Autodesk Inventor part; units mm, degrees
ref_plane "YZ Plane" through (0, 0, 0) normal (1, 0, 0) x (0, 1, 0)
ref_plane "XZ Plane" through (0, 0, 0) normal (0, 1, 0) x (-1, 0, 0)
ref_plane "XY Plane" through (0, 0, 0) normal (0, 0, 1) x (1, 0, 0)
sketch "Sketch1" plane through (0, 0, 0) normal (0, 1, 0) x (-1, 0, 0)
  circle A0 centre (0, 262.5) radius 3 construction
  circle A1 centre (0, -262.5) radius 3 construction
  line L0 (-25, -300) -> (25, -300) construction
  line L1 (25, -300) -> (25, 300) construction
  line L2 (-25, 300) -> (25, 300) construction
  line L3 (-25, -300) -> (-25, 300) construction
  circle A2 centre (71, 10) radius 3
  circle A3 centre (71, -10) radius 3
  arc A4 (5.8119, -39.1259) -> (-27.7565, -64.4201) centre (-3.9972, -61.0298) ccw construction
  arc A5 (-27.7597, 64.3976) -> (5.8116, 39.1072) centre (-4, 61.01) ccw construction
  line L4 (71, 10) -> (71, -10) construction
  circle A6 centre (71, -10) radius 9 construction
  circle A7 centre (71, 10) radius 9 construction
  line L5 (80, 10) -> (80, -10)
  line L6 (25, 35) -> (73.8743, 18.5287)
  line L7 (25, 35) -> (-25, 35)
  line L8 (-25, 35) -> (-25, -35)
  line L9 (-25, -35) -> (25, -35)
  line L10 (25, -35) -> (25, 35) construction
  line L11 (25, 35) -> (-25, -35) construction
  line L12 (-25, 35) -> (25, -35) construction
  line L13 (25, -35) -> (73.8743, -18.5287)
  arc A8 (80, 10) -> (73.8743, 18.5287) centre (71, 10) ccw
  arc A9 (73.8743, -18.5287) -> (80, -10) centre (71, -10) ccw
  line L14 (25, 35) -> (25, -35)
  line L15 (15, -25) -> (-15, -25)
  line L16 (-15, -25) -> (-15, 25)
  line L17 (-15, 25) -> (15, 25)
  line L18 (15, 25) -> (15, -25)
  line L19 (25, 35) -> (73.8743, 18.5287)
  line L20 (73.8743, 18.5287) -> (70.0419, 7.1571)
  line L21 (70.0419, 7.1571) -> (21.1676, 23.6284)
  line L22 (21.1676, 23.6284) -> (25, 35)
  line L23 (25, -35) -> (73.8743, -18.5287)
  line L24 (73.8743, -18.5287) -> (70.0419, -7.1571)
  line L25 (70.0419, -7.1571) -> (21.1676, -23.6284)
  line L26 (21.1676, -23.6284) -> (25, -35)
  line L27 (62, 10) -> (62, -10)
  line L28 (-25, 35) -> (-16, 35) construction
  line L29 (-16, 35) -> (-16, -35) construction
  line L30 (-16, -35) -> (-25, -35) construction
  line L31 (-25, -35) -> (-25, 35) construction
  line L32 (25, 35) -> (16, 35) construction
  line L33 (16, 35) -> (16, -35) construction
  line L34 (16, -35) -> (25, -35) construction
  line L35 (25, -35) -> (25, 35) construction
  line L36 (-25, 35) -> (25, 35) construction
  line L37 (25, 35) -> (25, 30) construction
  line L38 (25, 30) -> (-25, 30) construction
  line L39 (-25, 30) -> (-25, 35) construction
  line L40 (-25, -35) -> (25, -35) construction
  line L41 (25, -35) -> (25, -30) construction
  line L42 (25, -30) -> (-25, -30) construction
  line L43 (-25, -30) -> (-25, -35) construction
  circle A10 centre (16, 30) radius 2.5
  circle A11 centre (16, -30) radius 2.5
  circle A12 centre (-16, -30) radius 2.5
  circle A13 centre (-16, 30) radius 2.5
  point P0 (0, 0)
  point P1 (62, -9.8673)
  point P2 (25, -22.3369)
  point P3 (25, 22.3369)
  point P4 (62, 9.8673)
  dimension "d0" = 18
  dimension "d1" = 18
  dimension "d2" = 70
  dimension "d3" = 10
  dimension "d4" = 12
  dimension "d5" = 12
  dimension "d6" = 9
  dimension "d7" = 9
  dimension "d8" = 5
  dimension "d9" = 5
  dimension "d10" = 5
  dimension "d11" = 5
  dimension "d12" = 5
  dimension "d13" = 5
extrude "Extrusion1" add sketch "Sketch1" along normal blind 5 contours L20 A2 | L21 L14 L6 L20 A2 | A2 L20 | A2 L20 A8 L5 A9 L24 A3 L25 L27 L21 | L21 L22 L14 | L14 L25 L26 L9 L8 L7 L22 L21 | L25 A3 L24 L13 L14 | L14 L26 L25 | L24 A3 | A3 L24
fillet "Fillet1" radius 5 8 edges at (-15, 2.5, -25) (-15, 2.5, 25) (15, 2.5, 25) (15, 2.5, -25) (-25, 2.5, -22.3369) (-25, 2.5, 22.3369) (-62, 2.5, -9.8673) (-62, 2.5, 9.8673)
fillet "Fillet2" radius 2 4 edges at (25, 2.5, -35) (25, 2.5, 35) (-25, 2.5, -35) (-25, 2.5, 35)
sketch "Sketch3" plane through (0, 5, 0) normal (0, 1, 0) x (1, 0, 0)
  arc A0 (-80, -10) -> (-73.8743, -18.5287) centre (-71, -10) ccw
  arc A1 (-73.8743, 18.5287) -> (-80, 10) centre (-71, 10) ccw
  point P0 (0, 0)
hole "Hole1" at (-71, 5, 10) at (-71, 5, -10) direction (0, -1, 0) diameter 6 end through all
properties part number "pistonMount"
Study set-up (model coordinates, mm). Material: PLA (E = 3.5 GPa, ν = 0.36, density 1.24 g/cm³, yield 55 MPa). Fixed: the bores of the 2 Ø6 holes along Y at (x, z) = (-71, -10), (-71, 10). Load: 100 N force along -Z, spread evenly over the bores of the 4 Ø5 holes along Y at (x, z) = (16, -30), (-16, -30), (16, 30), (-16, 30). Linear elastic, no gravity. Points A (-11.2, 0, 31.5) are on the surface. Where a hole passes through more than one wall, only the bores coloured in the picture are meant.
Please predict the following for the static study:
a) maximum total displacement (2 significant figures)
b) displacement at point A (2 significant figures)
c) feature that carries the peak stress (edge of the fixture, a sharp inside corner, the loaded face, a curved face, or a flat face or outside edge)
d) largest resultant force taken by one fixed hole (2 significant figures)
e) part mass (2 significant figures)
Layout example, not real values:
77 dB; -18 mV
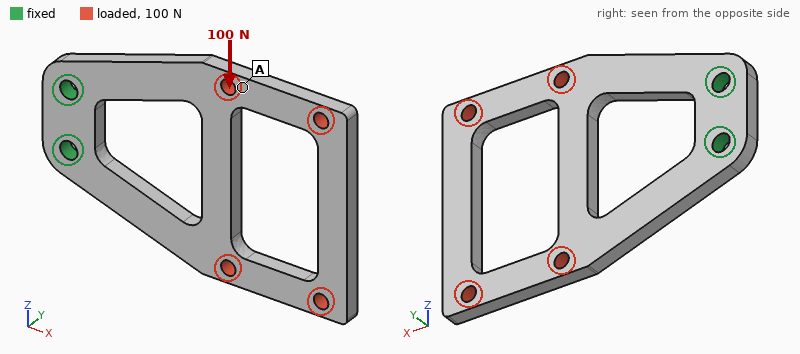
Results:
1.3 mm; 0.79 mm; a curved face; 220 N; 22 g
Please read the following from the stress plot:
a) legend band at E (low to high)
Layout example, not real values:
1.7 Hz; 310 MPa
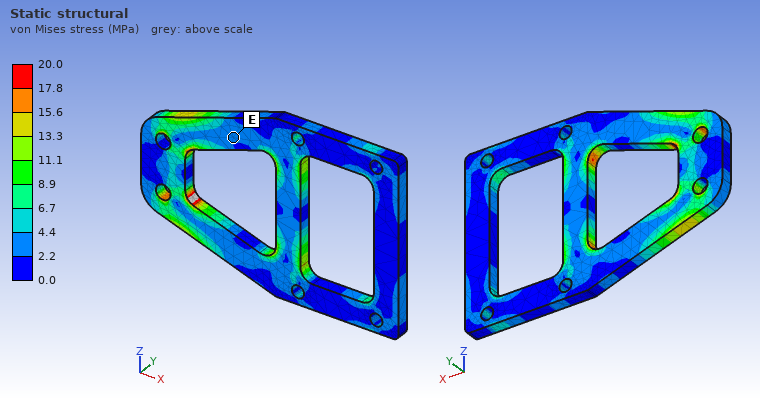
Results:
2.2 to 4.4 MPa
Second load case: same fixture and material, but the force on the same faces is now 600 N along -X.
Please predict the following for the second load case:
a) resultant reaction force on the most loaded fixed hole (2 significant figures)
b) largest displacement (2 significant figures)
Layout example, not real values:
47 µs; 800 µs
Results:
310 N; 0.15 mm
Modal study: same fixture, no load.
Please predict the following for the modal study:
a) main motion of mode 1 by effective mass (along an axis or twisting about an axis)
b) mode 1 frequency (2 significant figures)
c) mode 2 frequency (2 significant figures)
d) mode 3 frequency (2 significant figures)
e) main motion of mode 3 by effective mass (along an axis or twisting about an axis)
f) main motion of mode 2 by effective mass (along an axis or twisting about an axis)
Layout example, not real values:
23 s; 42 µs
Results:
along Y; 120 Hz; 290 Hz; 440 Hz; along Z; twisting about X
